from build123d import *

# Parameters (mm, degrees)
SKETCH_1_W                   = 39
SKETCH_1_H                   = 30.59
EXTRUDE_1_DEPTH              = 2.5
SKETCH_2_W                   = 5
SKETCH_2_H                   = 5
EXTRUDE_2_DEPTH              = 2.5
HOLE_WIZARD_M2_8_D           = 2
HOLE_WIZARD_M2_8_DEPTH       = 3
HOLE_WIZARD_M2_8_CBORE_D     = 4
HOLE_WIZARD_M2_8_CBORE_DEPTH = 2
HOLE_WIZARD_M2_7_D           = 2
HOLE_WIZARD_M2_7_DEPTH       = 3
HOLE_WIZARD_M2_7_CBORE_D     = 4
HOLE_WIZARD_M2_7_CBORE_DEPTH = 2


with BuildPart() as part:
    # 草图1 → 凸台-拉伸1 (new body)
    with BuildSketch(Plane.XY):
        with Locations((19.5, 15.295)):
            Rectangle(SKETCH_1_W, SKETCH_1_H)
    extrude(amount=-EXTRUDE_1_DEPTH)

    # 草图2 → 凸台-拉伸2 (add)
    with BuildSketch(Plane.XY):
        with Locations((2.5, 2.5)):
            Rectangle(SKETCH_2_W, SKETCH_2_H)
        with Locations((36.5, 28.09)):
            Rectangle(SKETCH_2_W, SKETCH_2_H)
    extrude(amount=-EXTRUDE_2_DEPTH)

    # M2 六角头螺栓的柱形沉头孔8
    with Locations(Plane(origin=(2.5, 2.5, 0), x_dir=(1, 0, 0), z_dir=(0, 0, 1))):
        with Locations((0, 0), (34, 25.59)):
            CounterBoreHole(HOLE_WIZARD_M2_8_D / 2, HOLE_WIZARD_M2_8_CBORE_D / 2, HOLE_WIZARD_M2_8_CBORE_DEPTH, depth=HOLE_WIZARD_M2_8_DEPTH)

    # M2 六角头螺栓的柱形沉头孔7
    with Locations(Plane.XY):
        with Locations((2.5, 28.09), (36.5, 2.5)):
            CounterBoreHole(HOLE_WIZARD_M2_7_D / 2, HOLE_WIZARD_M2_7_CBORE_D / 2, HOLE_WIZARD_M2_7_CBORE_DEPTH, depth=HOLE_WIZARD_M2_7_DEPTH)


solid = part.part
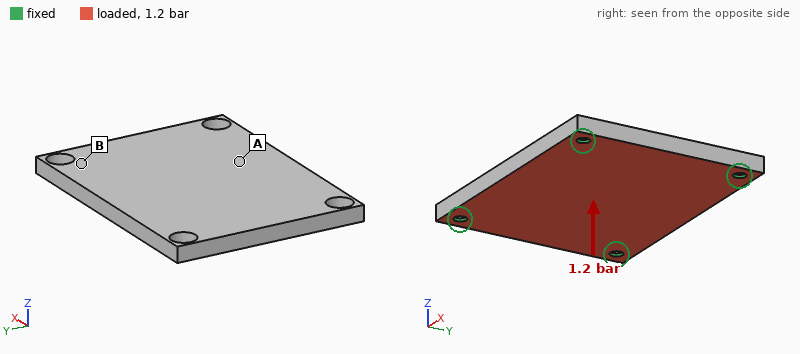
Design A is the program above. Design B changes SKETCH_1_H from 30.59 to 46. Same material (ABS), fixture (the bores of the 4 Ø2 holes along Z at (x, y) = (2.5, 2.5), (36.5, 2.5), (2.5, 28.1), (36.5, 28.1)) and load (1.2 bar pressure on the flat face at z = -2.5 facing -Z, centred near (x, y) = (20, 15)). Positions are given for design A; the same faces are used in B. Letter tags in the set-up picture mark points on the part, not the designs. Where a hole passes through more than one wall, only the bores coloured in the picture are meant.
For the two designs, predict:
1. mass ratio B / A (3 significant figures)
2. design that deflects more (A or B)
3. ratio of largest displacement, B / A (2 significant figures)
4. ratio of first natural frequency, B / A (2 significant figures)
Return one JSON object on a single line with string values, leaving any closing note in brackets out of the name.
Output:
{"mass ratio B / A": "1.52", "design that deflects more": "B", "ratio of largest displacement, B / A": "1.3", "ratio of first natural frequency, B / A": "0.93"}
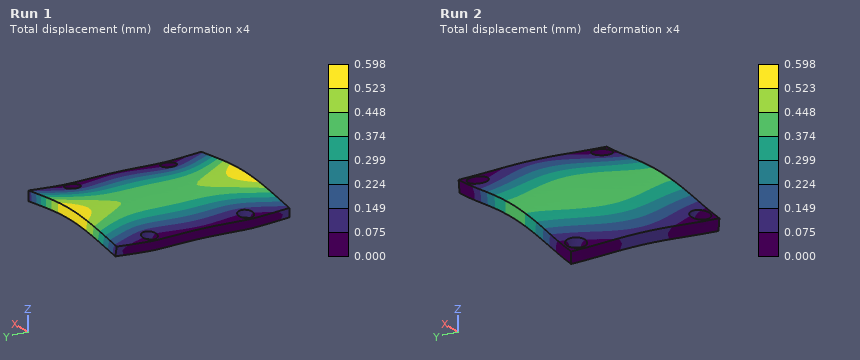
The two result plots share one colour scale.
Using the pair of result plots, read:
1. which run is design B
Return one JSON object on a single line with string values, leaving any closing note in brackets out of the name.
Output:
{"which run is design B": "Run 1"}
